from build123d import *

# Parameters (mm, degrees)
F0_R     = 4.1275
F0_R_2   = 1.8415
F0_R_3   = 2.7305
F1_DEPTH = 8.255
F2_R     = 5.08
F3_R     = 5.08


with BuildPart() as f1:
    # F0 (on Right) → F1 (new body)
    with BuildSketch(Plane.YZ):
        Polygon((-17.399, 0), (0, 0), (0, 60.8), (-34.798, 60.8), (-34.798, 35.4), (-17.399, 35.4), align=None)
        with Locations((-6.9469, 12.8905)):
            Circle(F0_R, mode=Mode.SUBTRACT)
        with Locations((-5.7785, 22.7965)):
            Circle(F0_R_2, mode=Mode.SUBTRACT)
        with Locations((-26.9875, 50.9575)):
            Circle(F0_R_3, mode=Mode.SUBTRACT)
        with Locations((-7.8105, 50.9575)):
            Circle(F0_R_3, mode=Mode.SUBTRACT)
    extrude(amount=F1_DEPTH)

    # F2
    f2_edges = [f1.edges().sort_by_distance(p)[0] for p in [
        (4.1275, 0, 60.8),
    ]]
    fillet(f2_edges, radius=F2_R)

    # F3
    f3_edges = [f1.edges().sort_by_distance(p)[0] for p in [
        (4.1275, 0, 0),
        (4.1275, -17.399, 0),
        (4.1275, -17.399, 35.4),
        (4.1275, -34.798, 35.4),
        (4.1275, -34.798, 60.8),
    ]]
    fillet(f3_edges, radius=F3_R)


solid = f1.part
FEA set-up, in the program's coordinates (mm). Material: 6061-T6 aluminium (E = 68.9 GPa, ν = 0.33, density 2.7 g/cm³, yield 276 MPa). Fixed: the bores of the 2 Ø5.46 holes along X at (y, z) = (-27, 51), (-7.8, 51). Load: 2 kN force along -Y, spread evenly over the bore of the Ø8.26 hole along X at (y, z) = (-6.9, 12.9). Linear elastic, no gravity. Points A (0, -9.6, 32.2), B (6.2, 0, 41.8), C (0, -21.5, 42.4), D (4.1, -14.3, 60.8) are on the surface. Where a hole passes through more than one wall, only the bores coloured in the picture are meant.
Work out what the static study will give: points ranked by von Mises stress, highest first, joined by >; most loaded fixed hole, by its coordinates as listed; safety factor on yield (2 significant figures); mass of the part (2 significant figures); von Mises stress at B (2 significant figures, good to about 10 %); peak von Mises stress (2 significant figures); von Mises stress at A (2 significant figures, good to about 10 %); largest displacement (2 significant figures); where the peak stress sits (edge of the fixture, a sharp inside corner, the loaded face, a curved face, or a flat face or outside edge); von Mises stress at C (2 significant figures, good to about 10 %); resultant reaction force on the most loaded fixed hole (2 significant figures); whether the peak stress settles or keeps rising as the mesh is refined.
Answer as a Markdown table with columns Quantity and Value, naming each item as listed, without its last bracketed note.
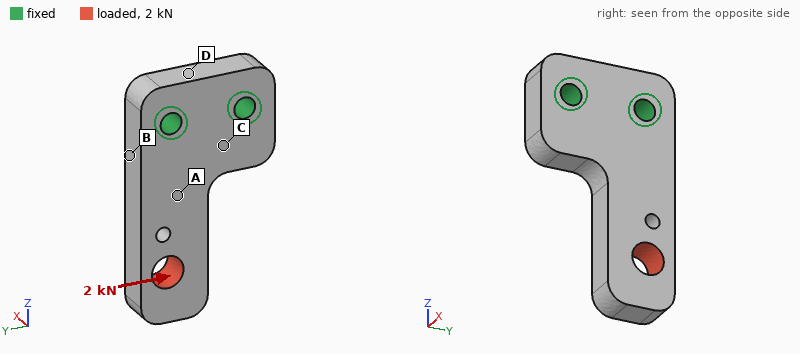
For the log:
| Quantity | Value |
|---|---|
| points ranked by von Mises stress, highest first, joined by > | B > C > A > D |
| most loaded fixed hole, by its coordinates as listed | (-27, 51) |
| safety factor on yield | 1.6 |
| mass of the part | 30 g |
| von Mises stress at B | 70 MPa |
| peak von Mises stress | 170 MPa |
| von Mises stress at A | 30 MPa |
| largest displacement | 0.15 mm |
| where the peak stress sits | a curved face |
| von Mises stress at C | 52 MPa |
| resultant reaction force on the most loaded fixed hole | 3.8 kN |
| whether the peak stress settles or keeps rising as the mesh is refined | settles |
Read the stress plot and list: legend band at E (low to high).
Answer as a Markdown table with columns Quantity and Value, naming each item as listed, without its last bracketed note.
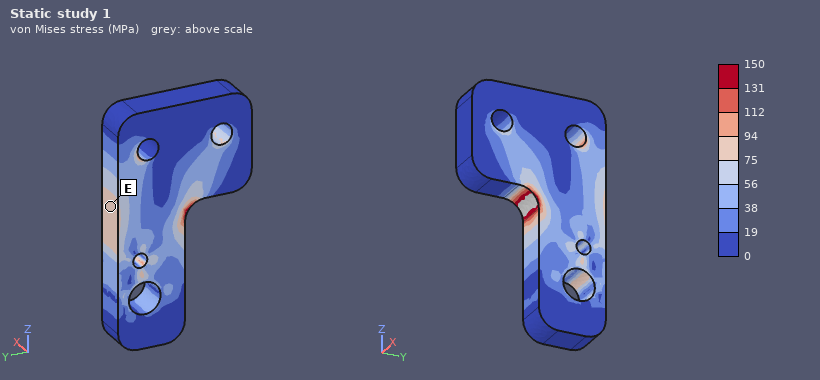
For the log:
| Quantity | Value |
|---|---|
| legend band at E | 75 to 94 MPa |
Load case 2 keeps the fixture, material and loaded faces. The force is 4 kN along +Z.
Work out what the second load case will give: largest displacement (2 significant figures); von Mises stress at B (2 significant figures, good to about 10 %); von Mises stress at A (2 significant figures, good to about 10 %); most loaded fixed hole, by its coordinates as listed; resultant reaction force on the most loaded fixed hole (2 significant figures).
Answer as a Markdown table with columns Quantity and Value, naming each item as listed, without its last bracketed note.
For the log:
| Quantity | Value |
|---|---|
| largest displacement | 49 µm |
| von Mises stress at B | 37 MPa |
| von Mises stress at A | 26 MPa |
| most loaded fixed hole, by its coordinates as listed | (-7.8, 51) |
| resultant reaction force on the most loaded fixed hole | 3.9 kN |
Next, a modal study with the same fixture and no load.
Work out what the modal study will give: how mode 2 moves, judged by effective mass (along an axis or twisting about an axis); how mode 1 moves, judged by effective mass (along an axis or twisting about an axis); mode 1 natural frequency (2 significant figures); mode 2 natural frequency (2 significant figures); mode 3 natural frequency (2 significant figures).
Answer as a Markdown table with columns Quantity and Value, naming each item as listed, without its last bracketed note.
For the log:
| Quantity | Value |
|---|---|
| how mode 2 moves, judged by effective mass | along Y |
| how mode 1 moves, judged by effective mass | along X |
| mode 1 natural frequency | 3200 Hz |
| mode 2 natural frequency | 7300 Hz |
| mode 3 natural frequency | 13 kHz |
